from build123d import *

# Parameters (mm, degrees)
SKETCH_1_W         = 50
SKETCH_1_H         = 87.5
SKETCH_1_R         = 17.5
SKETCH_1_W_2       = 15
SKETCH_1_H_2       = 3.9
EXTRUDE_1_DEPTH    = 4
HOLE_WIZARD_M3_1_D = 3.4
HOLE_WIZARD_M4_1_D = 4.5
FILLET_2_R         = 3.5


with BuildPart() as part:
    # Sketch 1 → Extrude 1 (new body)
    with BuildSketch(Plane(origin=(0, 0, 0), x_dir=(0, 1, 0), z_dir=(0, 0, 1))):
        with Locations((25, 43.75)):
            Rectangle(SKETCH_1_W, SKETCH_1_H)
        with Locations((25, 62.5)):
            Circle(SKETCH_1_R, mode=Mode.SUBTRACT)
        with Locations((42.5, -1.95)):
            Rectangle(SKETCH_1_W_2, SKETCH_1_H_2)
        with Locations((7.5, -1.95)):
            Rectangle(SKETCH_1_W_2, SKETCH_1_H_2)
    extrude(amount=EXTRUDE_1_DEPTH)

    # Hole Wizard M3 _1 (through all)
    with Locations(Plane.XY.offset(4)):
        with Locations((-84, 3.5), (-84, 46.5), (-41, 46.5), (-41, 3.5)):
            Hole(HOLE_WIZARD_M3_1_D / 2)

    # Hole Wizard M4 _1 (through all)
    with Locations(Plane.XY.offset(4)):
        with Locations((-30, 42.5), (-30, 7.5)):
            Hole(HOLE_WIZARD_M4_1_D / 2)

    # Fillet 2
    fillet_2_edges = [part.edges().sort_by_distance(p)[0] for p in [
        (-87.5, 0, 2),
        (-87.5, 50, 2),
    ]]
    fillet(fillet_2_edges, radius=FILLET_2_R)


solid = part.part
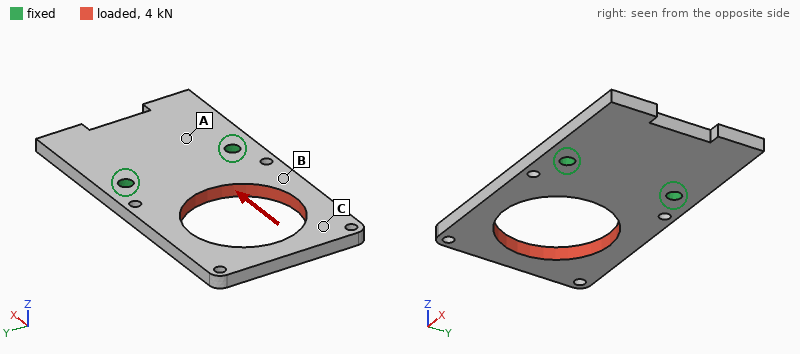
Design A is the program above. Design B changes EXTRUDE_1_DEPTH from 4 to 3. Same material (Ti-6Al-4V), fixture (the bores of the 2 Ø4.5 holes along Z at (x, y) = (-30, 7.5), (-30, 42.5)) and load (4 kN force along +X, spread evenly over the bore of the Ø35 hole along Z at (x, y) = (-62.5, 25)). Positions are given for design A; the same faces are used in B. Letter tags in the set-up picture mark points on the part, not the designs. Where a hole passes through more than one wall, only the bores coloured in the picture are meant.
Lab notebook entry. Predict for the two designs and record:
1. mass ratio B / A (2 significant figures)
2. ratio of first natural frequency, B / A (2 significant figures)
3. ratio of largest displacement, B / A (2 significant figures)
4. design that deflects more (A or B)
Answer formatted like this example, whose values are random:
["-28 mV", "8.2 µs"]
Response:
["0.75", "0.76", "1.3", "B"]
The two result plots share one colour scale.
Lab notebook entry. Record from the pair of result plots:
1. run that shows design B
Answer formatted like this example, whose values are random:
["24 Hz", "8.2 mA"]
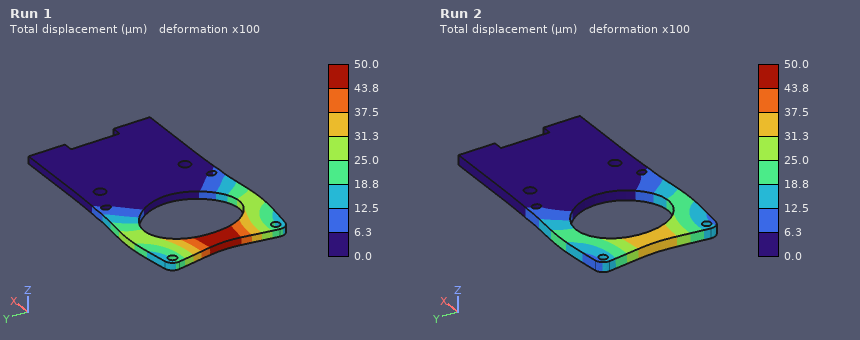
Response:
["Run 1"]
